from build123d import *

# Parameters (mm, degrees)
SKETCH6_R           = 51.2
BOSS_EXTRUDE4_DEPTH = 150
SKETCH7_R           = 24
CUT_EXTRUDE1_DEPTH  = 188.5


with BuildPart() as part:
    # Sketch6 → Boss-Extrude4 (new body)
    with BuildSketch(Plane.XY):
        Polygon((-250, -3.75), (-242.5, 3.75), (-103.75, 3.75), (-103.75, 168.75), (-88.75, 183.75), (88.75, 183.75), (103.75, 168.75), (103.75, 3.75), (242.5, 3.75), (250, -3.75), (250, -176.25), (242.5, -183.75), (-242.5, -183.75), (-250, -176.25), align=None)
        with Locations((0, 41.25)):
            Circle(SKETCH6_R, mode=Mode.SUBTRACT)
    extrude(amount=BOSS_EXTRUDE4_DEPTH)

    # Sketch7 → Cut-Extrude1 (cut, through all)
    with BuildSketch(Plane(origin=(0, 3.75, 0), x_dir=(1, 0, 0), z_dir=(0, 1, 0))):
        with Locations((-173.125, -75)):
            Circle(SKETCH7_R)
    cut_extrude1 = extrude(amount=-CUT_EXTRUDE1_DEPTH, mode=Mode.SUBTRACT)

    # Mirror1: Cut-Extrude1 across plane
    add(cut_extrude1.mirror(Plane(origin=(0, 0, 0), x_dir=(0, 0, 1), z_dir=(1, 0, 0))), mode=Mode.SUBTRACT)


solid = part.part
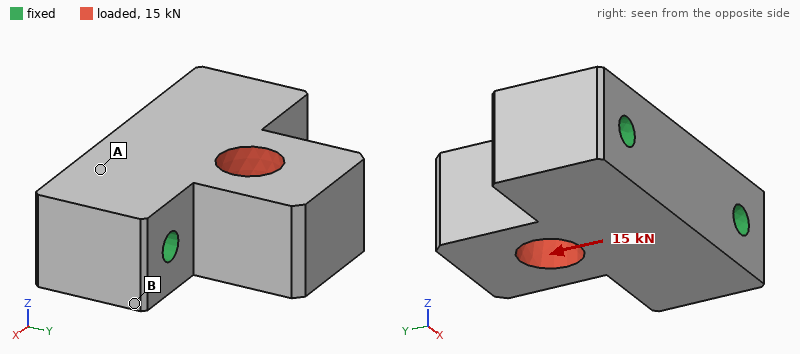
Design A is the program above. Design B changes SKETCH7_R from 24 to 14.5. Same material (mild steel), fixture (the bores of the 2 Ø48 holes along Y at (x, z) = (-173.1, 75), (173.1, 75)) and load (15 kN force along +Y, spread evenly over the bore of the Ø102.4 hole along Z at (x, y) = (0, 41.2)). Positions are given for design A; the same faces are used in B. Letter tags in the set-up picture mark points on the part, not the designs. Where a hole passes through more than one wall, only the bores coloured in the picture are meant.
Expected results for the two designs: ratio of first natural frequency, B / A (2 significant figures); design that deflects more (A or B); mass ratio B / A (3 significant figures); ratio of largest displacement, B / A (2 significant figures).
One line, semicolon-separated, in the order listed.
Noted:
0.94; B; 1.02; 1.1
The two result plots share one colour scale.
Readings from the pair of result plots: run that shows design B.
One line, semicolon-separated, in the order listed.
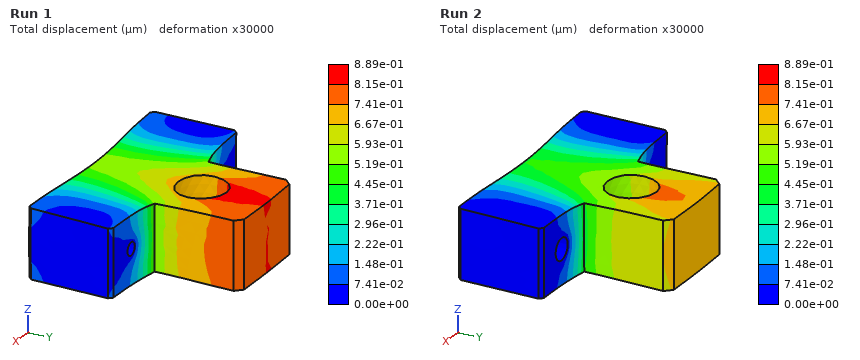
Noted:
Run 1
